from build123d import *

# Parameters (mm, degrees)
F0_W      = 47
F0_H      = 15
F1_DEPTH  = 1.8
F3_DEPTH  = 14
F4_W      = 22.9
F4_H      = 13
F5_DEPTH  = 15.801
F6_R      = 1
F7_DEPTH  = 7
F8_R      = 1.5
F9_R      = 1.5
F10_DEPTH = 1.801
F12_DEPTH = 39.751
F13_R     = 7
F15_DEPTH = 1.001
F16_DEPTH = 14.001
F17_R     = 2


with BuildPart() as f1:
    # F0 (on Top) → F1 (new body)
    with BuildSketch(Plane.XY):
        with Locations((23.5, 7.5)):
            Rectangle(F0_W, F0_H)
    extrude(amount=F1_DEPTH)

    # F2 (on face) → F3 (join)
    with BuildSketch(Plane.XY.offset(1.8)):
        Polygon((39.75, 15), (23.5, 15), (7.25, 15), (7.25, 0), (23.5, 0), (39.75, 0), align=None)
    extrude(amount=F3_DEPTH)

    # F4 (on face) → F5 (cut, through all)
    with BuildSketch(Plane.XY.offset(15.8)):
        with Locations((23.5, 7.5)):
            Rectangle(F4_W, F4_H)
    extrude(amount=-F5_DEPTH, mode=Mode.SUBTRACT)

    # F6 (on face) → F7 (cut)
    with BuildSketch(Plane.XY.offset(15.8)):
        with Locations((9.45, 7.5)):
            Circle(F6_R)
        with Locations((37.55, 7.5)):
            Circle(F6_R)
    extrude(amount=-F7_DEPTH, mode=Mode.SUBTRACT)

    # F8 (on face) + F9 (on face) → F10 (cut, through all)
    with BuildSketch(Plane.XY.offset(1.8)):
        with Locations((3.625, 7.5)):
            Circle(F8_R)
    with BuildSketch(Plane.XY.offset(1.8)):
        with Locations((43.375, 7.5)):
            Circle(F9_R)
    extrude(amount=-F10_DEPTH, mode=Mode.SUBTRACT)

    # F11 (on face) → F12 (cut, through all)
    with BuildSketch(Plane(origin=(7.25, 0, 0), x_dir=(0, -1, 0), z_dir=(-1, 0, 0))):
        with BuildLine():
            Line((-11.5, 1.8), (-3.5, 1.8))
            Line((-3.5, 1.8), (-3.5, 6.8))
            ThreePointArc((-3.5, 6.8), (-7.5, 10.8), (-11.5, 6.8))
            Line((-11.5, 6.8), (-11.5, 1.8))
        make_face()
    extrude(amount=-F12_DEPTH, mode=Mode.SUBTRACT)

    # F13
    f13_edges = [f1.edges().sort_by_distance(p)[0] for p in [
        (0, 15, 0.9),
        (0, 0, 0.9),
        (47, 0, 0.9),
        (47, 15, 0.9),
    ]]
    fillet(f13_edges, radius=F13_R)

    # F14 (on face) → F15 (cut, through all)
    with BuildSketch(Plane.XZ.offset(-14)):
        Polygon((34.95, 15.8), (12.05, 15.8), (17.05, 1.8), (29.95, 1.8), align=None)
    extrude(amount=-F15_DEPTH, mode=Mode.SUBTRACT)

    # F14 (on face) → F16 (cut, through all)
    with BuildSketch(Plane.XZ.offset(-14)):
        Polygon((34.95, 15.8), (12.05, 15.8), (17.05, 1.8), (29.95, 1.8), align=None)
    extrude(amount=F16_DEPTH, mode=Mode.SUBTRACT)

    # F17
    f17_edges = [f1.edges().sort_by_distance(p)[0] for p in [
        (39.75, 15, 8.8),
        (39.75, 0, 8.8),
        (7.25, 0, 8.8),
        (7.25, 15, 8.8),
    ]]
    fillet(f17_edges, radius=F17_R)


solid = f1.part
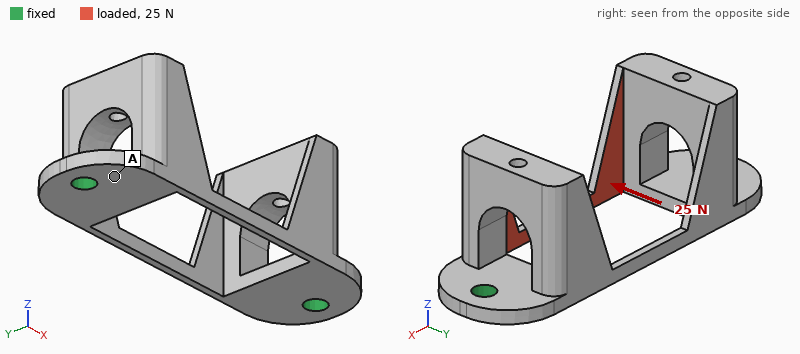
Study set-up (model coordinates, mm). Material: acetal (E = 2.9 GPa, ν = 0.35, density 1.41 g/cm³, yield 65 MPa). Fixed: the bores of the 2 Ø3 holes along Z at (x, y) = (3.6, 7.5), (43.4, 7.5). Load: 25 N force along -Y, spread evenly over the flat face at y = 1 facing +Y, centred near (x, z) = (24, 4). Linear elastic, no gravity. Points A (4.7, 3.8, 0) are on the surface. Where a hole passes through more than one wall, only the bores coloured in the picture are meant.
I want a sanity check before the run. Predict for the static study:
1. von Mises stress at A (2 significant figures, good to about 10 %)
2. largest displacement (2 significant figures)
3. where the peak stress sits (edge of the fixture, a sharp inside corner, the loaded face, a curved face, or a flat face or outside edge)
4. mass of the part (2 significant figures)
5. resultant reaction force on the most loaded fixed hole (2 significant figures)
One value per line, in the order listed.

2.9 MPa
0.51 mm
a flat face or outside edge
2.9 g
13 N
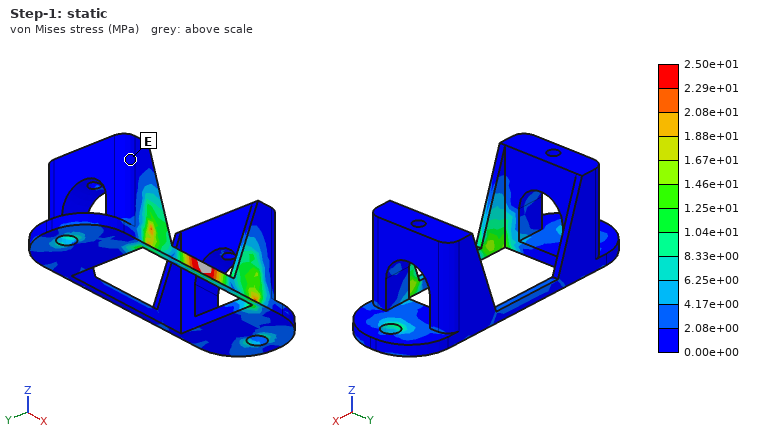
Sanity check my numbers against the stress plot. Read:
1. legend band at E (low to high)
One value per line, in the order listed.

0.00e+00 to 2.08e+00 MPa
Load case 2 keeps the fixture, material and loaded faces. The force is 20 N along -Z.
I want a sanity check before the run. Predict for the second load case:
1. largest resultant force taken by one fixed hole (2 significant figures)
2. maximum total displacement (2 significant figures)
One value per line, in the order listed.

10 N
0.38 mm
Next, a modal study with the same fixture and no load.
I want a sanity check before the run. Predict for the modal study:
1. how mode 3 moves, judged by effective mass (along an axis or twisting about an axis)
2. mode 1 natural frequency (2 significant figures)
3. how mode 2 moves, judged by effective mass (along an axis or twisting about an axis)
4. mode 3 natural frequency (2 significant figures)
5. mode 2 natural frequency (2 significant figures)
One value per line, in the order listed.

twisting about Z
950 Hz
along Y
1300 Hz
1300 Hz
